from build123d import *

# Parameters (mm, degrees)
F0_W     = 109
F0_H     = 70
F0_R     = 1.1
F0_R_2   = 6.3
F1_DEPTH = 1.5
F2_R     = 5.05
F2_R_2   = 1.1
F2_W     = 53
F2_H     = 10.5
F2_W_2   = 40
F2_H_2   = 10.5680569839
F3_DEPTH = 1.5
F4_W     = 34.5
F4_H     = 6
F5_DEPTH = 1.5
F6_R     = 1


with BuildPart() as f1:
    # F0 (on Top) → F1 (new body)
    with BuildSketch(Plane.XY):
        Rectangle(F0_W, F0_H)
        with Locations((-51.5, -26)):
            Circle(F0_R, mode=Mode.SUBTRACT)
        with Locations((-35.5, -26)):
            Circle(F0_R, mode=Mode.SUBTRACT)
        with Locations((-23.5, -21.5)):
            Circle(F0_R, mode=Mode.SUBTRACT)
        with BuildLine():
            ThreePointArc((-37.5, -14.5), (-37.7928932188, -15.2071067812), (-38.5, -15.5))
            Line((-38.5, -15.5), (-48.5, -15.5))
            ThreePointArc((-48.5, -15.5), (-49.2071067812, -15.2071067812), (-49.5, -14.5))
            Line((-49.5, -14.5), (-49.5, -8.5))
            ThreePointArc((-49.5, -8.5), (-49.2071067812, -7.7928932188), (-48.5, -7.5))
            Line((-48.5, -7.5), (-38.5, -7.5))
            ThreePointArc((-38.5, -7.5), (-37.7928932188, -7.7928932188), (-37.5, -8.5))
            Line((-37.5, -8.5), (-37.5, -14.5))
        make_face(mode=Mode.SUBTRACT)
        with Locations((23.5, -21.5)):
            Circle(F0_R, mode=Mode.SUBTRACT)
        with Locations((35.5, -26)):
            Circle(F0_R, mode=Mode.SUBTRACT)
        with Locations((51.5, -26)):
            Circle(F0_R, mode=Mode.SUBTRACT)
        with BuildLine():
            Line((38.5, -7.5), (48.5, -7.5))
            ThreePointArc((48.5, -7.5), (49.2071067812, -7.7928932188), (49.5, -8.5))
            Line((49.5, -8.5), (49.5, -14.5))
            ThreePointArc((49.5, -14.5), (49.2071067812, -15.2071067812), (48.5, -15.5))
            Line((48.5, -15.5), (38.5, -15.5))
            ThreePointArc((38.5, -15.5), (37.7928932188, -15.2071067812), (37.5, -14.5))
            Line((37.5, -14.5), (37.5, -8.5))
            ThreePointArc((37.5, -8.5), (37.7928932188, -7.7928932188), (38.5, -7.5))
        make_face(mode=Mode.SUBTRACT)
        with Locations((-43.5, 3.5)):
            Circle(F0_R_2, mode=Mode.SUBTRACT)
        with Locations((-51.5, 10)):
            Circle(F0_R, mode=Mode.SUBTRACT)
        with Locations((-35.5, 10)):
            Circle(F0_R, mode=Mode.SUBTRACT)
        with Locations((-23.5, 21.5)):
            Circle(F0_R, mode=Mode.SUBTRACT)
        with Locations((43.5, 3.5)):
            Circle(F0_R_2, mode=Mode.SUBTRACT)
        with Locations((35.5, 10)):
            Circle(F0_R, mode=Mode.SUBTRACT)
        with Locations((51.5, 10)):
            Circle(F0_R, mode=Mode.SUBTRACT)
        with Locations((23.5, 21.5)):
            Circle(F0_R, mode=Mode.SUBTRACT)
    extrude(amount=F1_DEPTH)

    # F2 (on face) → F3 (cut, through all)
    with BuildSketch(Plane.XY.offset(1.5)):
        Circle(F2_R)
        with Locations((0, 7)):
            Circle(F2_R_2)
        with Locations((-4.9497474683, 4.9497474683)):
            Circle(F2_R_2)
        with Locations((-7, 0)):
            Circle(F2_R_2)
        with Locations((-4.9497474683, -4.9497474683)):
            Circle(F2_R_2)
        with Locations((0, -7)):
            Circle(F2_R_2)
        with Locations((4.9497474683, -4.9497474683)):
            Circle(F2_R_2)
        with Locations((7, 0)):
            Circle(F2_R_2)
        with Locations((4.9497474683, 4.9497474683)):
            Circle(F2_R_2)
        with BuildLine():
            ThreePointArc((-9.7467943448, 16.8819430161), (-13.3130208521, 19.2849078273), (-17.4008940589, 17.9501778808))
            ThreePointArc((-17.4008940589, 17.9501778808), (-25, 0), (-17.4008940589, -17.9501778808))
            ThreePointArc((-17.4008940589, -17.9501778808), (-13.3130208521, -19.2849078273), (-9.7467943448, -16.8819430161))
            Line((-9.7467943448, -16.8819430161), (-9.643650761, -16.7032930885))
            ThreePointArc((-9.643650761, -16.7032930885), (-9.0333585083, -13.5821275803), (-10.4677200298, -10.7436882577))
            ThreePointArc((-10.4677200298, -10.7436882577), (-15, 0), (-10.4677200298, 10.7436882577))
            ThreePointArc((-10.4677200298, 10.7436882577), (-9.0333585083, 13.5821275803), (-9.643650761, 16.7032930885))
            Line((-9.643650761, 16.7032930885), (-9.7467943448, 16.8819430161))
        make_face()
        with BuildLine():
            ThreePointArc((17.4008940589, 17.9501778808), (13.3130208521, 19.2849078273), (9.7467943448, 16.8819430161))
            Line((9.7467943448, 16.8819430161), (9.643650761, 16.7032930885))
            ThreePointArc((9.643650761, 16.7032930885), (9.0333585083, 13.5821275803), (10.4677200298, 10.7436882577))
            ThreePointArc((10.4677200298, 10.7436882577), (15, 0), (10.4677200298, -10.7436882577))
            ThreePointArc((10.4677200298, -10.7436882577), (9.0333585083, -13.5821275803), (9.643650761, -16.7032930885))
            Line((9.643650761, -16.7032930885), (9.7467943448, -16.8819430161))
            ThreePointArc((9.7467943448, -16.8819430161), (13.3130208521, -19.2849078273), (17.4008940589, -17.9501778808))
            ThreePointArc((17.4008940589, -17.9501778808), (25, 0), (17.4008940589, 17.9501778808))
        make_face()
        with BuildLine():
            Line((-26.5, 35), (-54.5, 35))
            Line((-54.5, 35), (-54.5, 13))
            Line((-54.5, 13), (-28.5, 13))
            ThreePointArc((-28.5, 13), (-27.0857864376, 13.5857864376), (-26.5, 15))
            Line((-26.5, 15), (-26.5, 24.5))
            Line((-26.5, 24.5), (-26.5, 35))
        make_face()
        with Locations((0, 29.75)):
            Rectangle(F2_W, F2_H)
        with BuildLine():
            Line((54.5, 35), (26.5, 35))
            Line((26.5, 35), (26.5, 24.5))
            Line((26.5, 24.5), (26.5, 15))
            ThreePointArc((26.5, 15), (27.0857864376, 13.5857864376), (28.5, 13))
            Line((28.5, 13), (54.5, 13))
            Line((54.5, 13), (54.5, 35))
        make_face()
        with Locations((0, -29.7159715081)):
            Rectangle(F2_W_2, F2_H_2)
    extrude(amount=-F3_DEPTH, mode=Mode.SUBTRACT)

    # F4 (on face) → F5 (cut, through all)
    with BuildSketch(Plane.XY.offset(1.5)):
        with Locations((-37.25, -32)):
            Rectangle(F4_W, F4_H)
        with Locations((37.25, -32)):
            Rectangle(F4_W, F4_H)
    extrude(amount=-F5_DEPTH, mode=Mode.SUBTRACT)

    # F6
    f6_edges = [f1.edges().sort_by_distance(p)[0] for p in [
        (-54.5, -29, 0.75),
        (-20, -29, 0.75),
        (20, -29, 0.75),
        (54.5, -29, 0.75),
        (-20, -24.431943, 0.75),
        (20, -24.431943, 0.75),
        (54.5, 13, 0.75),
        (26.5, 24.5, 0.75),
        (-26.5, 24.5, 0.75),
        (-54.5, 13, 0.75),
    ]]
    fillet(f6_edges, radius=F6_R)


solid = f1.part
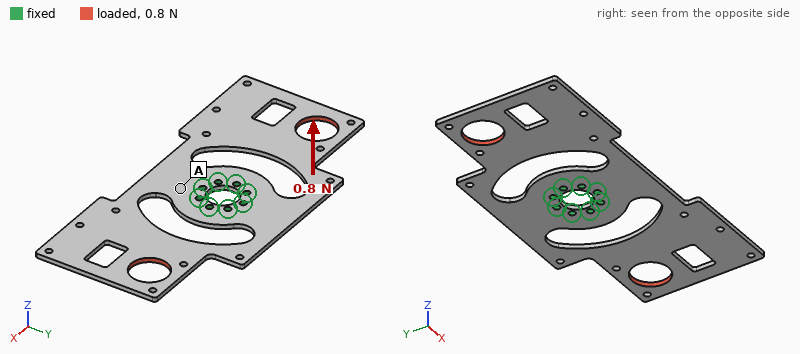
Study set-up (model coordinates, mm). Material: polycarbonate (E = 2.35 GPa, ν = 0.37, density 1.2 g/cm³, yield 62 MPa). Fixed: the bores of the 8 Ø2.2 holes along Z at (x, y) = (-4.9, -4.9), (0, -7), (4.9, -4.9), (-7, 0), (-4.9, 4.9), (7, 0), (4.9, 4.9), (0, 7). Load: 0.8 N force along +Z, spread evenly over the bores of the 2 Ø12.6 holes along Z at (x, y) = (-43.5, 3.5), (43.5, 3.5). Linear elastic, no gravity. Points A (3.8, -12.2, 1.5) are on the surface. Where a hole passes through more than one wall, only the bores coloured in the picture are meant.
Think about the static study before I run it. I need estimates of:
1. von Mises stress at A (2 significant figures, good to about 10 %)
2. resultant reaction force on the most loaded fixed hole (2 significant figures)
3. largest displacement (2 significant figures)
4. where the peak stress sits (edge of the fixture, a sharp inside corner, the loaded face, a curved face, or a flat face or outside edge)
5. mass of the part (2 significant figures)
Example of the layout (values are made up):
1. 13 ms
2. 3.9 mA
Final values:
1. 0.70 MPa
2. 0.43 N
3. 1.4 mm
4. a curved face
5. 6.5 g
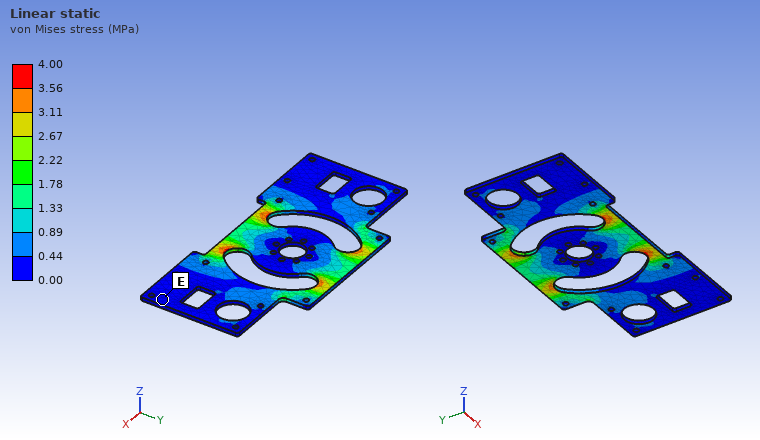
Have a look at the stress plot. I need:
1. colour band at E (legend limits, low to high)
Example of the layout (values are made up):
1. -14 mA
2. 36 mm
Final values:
1. 0.00 to 0.44 MPa
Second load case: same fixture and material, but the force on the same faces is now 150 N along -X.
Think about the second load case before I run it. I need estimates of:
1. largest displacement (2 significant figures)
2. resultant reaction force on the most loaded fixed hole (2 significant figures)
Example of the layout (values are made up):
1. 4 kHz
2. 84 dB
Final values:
1. 0.43 mm
2. 55 N
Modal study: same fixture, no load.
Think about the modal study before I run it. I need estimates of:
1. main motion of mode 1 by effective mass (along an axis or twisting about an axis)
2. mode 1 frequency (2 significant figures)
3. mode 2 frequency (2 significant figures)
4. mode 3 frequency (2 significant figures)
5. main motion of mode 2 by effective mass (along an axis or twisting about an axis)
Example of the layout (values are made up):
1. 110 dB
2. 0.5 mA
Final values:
1. twisting about Y
2. 75 Hz
3. 81 Hz
4. 260 Hz
5. along Z
